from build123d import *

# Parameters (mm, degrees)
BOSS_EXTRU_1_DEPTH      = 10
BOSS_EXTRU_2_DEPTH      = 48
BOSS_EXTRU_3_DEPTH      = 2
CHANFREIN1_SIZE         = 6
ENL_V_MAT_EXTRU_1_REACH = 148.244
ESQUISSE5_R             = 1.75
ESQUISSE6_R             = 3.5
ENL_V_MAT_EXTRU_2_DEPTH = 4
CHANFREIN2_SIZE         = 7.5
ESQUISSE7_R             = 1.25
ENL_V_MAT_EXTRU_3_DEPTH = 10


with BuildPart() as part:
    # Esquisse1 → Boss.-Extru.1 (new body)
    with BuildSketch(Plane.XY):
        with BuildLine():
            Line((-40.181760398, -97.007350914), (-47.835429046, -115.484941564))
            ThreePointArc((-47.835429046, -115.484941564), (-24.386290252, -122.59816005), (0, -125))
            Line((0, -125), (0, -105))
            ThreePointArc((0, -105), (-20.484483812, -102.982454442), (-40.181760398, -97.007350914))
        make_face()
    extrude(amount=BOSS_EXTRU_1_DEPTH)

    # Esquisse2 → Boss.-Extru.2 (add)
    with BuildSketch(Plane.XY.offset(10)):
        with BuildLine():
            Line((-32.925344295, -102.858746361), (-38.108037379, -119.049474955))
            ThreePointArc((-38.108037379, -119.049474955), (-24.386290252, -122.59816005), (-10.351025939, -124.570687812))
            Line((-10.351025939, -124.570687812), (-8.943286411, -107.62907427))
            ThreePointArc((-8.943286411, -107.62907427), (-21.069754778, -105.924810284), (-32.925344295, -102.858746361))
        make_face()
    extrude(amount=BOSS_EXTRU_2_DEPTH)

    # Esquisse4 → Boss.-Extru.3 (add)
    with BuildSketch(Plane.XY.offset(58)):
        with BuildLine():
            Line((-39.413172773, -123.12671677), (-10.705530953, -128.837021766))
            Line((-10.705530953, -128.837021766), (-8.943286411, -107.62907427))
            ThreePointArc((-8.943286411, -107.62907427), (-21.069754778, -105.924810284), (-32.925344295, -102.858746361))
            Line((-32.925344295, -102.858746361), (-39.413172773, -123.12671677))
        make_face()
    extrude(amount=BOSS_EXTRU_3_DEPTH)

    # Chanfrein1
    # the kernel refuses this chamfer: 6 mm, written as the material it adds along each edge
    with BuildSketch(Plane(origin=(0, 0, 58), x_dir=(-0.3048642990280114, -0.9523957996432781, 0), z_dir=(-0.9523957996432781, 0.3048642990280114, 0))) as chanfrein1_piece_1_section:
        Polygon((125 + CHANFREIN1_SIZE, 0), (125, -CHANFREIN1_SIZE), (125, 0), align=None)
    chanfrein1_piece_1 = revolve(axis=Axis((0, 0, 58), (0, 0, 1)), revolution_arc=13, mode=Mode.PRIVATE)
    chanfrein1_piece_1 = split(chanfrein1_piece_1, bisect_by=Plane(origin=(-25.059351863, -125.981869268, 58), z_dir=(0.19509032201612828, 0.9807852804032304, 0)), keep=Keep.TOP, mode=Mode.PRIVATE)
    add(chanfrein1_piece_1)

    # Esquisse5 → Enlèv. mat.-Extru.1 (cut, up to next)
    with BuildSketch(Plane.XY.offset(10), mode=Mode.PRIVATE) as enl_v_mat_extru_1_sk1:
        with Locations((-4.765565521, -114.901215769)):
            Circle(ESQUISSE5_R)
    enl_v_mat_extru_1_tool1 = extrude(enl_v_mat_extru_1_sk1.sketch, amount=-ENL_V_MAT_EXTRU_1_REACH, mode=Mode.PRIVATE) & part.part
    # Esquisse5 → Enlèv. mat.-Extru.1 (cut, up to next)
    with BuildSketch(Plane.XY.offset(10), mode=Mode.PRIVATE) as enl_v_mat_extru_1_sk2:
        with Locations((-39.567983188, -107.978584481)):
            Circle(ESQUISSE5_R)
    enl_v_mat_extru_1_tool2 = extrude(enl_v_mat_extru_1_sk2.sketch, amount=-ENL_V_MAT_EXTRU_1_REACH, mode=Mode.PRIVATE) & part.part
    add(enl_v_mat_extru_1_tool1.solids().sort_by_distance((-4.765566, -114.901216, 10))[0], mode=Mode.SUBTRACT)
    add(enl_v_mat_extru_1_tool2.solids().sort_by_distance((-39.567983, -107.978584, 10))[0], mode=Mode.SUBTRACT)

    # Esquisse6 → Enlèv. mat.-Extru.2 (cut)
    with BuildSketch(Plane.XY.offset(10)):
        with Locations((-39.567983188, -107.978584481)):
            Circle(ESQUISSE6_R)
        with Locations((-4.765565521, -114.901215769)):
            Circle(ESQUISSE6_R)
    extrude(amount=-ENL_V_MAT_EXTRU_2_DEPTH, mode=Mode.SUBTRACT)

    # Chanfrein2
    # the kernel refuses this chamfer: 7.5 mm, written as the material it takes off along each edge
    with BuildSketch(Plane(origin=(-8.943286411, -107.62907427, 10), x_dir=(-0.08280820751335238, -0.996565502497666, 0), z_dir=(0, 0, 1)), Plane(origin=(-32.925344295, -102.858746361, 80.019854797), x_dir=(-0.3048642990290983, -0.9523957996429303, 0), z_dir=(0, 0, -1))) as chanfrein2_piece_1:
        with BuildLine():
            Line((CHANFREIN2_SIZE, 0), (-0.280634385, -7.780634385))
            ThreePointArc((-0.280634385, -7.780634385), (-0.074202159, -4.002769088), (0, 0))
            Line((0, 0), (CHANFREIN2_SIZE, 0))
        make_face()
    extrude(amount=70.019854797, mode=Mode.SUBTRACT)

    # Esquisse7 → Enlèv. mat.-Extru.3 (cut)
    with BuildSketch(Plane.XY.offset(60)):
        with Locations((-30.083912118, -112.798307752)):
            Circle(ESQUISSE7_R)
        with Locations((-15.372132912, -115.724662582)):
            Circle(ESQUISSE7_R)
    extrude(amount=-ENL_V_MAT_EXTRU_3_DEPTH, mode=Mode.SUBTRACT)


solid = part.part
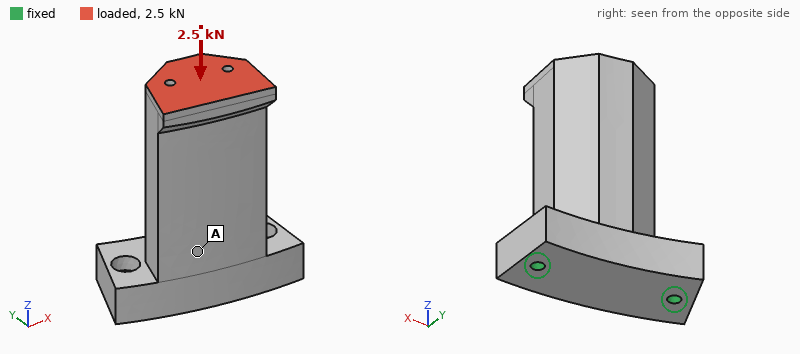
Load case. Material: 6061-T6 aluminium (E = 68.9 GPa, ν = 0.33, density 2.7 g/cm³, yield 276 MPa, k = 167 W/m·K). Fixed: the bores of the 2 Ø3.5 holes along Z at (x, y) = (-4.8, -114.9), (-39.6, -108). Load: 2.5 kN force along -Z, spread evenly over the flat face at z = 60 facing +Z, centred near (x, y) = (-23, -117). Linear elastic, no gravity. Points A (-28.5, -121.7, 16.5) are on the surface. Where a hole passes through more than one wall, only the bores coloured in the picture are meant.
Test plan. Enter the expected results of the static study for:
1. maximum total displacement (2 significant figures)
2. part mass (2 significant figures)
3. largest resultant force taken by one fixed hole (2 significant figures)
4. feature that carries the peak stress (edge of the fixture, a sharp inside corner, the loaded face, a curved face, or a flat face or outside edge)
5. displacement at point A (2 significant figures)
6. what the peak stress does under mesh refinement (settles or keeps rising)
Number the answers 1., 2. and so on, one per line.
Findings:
1. 89 µm
2. 78 g
3. 1.4 kN
4. edge of the fixture
5. 27 µm
6. keeps rising
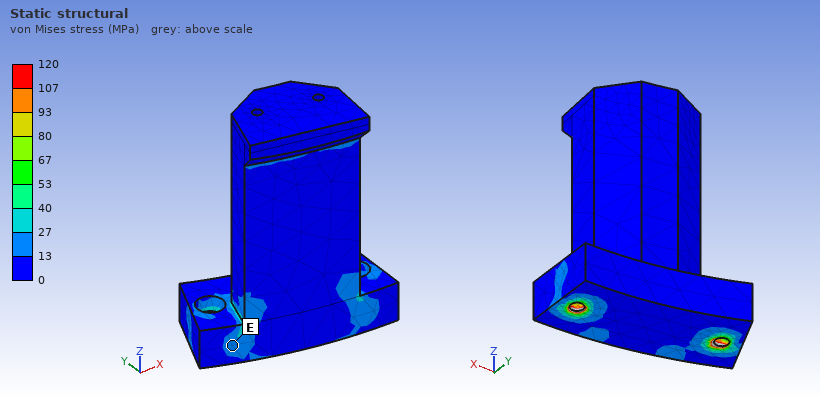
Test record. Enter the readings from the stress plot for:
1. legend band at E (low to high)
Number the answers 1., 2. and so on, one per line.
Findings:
1. 13 to 27 MPa
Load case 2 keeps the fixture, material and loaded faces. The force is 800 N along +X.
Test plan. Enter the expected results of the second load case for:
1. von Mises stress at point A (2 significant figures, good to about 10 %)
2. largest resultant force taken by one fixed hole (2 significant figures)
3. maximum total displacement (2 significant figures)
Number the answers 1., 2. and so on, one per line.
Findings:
1. 9.9 MPa
2. 1.4 kN
3. 87 µm
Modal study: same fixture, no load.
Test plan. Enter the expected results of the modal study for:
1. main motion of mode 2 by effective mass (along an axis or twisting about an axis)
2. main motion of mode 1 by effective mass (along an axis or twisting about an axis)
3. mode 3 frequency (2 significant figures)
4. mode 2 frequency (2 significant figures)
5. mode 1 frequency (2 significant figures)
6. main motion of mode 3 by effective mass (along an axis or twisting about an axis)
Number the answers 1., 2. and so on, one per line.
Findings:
1. along X
2. along Y
3. 11 kHz
4. 4600 Hz
5. 1800 Hz
6. along Z
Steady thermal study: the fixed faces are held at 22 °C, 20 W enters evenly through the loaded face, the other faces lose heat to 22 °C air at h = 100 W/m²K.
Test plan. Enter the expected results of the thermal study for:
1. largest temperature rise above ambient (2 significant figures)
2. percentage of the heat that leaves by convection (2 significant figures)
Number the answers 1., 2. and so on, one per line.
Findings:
1. 17 K
2. 25 %
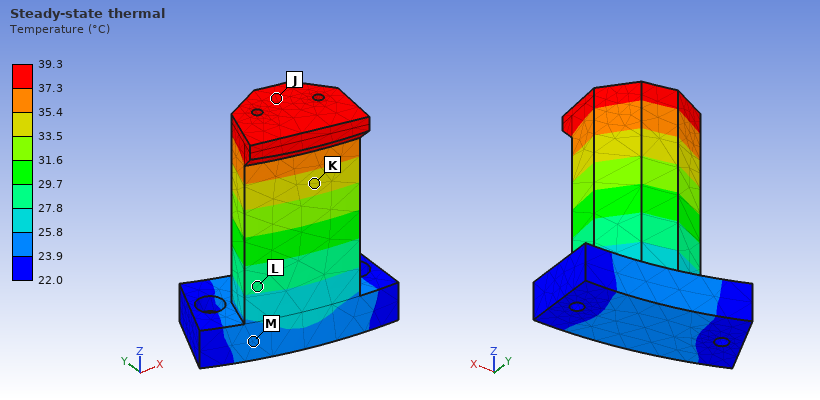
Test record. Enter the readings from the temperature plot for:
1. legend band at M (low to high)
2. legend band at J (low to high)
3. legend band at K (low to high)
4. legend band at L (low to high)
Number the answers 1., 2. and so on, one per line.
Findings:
1. 23.9 to 25.8 °C
2. 37.3 to 39.3 °C
3. 33.5 to 35.4 °C
4. 27.8 to 29.7 °C
